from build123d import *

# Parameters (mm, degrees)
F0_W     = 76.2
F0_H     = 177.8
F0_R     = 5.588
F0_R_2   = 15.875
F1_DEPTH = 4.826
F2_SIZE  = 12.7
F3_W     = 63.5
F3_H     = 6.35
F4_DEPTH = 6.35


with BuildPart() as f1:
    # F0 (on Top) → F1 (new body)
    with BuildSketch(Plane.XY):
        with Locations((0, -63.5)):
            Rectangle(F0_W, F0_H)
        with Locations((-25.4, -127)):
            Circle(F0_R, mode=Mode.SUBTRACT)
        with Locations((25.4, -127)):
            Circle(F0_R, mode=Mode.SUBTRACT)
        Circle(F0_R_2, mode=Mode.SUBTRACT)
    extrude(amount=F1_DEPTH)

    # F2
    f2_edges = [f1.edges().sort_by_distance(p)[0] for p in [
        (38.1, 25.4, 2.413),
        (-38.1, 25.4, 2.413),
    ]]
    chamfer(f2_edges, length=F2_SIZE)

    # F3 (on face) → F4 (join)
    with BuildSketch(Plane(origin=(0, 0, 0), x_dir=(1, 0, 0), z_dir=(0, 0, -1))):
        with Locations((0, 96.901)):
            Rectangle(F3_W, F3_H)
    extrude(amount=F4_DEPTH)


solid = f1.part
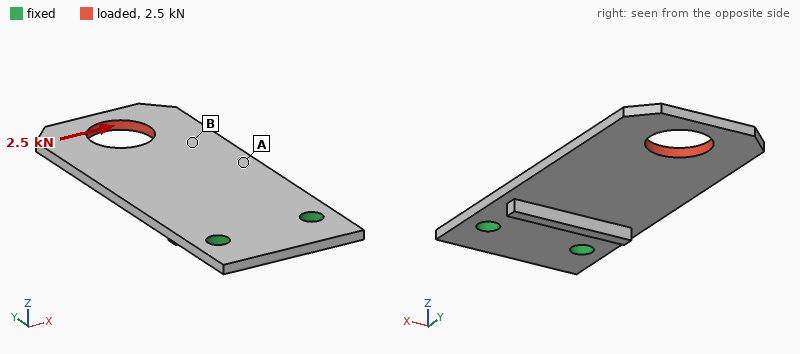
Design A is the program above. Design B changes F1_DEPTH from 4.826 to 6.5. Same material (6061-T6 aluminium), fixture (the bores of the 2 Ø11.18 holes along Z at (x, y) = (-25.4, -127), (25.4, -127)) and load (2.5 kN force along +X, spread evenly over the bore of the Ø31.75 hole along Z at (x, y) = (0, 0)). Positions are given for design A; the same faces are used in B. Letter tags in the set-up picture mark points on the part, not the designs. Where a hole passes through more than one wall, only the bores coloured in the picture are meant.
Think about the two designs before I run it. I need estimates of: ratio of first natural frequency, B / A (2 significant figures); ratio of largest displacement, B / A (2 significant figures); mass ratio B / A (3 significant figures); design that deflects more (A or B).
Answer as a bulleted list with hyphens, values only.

- 1.3
- 0.74
- 1.33
- A
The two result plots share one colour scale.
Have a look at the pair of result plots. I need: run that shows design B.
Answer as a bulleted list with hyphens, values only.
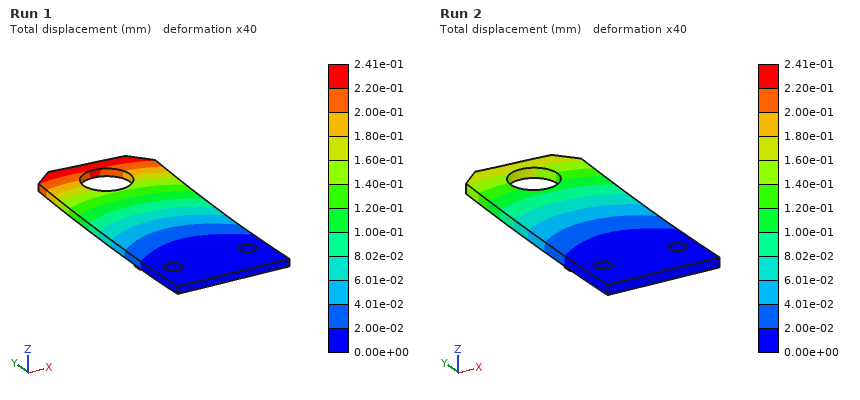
- Run 2
